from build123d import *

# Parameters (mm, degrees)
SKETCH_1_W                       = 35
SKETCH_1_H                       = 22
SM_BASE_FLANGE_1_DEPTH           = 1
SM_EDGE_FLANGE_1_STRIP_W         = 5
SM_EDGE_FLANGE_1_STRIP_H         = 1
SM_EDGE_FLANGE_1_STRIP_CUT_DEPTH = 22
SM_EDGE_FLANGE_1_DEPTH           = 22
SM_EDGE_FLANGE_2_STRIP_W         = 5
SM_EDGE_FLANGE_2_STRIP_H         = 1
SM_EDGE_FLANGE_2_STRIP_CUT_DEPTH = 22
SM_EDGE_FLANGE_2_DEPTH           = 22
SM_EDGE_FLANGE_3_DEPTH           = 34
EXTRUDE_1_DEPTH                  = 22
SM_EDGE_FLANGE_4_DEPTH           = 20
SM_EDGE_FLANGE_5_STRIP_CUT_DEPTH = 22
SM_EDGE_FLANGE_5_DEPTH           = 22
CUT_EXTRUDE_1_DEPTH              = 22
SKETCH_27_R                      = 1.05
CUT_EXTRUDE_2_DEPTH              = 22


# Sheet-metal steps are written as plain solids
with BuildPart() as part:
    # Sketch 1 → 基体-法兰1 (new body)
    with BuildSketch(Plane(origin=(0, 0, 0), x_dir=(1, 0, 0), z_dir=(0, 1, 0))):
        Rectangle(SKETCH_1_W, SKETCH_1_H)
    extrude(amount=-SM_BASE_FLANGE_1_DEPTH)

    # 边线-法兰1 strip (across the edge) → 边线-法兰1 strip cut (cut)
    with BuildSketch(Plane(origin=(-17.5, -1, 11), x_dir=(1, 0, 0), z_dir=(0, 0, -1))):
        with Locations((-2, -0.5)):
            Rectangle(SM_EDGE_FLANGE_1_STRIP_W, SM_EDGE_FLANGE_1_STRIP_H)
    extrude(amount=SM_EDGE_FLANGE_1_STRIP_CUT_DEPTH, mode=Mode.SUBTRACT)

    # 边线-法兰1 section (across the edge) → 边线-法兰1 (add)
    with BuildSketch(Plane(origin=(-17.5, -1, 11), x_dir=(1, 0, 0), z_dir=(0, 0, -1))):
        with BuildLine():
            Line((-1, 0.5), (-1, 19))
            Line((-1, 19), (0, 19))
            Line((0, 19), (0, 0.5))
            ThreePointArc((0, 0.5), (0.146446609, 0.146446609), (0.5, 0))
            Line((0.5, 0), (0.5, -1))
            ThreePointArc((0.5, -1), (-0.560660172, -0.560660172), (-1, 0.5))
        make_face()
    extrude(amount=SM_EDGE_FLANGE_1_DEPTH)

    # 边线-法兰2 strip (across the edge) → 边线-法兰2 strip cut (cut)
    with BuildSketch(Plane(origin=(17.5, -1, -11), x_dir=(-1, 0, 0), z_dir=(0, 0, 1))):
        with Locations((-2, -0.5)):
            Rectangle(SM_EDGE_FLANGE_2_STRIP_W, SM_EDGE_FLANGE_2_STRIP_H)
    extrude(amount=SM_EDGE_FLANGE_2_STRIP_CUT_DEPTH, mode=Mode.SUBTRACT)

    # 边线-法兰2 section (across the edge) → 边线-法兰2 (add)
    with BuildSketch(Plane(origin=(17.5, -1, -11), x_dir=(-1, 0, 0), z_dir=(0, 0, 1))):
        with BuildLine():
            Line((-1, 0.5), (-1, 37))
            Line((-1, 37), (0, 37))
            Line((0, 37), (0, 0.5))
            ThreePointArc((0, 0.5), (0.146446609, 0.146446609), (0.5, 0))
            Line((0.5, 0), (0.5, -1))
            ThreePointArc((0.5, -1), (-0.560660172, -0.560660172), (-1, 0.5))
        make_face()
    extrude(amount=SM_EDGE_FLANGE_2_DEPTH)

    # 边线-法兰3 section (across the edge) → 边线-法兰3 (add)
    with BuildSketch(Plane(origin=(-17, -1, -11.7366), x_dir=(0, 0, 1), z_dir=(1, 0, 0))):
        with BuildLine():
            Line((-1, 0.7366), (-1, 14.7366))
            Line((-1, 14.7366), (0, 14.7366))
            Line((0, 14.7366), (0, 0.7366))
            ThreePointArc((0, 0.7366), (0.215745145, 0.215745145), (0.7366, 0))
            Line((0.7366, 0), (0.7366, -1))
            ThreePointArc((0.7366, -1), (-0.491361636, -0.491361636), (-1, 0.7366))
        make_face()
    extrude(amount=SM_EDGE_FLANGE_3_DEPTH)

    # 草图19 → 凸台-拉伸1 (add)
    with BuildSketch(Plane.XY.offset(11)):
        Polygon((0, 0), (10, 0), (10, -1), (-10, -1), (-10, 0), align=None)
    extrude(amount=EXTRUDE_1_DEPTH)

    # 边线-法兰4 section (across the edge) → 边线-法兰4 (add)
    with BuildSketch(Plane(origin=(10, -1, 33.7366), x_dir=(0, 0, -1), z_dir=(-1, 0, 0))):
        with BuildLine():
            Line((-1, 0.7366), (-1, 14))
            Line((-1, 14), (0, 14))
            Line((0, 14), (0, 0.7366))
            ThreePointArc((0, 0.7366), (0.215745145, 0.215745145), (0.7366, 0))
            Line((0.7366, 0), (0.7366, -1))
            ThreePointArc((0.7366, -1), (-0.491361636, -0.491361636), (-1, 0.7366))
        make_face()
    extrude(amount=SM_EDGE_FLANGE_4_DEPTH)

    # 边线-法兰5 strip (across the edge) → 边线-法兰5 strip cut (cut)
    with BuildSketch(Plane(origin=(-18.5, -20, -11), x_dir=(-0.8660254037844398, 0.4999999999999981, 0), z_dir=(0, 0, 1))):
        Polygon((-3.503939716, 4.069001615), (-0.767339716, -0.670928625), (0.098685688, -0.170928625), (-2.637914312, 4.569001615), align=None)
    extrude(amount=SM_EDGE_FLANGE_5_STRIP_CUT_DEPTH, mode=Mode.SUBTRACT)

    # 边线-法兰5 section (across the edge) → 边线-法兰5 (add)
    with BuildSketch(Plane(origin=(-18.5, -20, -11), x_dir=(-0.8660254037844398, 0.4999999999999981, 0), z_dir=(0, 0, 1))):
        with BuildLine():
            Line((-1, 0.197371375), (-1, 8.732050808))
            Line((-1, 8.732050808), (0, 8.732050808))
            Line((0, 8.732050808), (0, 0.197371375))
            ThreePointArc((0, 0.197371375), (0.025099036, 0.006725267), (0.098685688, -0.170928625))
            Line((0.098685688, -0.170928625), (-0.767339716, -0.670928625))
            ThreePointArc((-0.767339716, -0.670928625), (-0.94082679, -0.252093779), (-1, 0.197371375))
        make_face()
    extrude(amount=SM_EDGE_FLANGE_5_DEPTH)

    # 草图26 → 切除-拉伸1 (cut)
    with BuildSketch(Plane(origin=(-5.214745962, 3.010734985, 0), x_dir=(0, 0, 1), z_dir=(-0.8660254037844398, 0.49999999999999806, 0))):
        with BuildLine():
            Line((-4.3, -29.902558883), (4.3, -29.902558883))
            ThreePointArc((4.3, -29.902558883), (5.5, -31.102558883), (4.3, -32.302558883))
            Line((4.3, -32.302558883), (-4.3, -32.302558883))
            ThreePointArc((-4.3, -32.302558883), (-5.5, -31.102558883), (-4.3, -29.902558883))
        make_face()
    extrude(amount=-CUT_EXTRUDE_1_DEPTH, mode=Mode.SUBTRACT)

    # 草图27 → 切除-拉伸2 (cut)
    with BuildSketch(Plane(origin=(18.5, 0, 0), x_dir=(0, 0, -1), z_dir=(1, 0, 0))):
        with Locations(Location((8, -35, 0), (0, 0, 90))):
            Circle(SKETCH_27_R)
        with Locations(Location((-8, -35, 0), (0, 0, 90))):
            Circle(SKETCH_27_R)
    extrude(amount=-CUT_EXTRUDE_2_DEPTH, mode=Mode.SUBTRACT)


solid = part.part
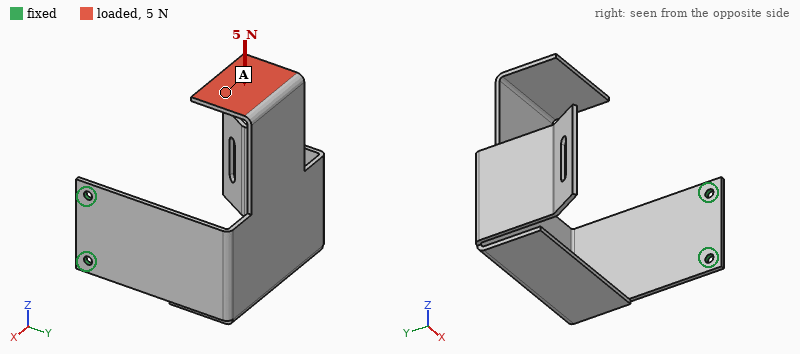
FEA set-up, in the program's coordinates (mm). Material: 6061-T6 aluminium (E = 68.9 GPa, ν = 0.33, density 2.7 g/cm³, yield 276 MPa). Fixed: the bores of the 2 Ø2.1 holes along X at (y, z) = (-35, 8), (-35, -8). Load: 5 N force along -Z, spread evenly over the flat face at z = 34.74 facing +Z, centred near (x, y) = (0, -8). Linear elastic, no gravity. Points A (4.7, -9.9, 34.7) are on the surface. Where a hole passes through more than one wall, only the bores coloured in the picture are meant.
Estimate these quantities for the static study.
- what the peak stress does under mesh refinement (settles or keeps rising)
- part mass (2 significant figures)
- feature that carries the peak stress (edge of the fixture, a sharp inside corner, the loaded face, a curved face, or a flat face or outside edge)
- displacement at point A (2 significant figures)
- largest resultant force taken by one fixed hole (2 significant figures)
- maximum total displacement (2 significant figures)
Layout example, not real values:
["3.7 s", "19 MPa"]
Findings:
["keeps rising", "9.4 g", "edge of the fixture", "0.59 mm", "9.9 N", "0.75 mm"]
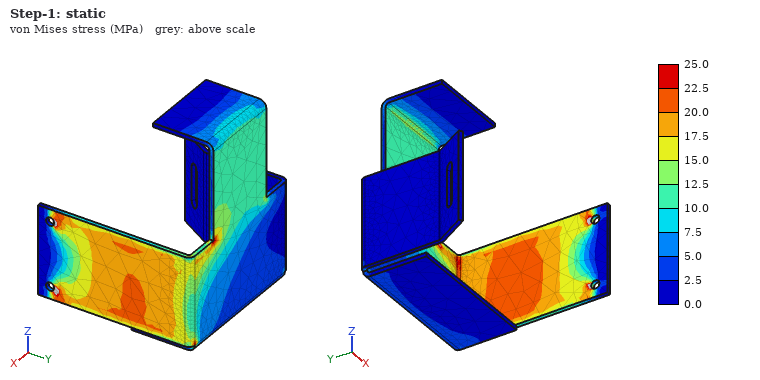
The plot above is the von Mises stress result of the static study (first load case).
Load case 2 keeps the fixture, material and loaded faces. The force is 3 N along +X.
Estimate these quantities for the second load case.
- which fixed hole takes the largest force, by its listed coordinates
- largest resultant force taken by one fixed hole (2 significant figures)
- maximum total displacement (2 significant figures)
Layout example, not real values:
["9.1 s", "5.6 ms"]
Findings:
["(-35, 8)", "7.7 N", "0.84 mm"]
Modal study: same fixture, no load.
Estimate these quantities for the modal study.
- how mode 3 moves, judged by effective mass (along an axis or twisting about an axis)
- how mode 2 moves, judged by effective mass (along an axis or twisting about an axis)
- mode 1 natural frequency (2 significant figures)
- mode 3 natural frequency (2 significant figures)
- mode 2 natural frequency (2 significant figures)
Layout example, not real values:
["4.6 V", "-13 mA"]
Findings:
["along X", "along Z", "120 Hz", "320 Hz", "170 Hz"]
